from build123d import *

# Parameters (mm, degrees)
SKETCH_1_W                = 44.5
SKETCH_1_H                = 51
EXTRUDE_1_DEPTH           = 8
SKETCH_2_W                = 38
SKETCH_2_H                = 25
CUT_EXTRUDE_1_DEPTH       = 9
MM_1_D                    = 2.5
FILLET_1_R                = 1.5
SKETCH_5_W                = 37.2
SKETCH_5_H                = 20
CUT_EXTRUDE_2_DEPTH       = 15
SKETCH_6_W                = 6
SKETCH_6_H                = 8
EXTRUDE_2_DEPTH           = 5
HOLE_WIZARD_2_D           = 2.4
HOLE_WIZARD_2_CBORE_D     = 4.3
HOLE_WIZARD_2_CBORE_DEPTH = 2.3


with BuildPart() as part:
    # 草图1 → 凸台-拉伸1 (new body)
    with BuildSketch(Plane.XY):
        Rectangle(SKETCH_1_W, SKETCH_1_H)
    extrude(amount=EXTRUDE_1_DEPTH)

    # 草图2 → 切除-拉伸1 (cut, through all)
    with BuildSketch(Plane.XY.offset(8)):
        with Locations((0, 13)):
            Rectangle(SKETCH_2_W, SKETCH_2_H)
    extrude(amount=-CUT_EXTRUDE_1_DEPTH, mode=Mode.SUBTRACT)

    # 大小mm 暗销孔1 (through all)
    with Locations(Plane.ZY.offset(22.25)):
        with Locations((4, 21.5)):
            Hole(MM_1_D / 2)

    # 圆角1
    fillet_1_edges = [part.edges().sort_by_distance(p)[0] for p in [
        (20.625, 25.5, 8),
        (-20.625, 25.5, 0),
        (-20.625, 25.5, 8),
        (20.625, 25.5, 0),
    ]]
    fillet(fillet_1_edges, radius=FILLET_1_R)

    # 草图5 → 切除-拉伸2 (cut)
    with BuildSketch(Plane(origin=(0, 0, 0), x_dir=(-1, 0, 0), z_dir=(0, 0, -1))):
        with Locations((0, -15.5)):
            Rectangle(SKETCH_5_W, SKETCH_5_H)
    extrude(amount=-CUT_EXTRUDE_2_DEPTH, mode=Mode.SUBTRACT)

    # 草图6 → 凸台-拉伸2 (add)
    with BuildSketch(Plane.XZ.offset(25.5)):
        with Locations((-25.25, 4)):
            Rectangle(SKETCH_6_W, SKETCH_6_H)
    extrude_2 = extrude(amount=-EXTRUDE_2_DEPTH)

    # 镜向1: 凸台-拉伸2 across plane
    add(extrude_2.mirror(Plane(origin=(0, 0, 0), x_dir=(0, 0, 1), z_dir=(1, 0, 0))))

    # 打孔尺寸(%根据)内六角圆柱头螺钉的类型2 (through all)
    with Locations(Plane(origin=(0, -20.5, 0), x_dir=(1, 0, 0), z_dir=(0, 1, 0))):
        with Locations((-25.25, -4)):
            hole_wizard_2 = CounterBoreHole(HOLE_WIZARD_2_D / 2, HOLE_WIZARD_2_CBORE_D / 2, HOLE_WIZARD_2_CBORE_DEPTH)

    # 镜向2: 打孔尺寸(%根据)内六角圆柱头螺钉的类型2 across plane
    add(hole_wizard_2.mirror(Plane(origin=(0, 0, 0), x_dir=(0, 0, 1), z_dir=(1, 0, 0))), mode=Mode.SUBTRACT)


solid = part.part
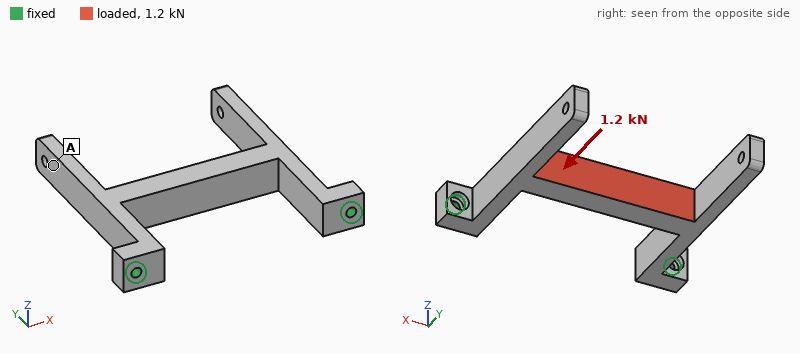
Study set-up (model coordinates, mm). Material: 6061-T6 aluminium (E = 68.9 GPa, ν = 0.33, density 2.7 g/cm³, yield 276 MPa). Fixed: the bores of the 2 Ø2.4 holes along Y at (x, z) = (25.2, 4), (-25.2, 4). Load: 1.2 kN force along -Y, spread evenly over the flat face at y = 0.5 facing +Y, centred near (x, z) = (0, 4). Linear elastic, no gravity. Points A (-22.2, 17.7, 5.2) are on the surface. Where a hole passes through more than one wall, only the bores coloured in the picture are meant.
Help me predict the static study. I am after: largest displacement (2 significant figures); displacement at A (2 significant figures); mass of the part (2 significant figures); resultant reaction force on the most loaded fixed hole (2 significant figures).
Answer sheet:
0.11 mm
0.081 mm
13 g
640 N
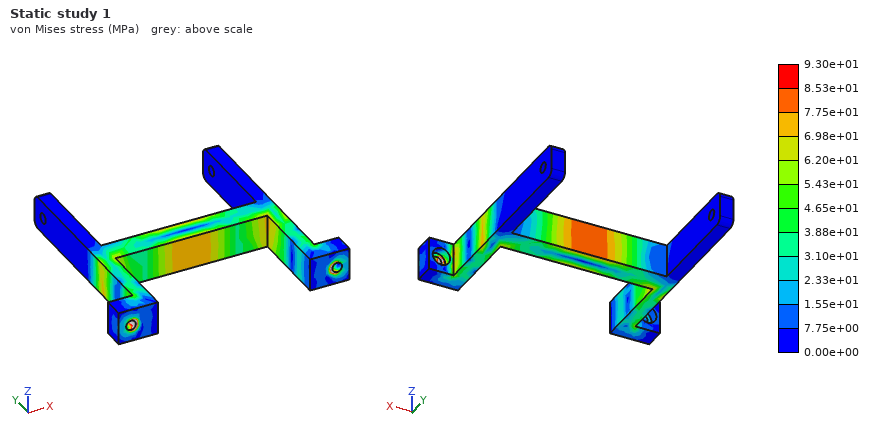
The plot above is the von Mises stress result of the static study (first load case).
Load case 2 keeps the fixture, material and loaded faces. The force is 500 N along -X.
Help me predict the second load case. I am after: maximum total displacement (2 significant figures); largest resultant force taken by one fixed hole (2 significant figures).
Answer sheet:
0.14 mm
310 N
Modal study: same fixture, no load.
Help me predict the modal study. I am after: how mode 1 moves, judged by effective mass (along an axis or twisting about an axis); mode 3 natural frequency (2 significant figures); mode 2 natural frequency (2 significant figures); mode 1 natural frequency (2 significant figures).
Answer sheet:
along Z
2800 Hz
2800 Hz
1700 Hz
